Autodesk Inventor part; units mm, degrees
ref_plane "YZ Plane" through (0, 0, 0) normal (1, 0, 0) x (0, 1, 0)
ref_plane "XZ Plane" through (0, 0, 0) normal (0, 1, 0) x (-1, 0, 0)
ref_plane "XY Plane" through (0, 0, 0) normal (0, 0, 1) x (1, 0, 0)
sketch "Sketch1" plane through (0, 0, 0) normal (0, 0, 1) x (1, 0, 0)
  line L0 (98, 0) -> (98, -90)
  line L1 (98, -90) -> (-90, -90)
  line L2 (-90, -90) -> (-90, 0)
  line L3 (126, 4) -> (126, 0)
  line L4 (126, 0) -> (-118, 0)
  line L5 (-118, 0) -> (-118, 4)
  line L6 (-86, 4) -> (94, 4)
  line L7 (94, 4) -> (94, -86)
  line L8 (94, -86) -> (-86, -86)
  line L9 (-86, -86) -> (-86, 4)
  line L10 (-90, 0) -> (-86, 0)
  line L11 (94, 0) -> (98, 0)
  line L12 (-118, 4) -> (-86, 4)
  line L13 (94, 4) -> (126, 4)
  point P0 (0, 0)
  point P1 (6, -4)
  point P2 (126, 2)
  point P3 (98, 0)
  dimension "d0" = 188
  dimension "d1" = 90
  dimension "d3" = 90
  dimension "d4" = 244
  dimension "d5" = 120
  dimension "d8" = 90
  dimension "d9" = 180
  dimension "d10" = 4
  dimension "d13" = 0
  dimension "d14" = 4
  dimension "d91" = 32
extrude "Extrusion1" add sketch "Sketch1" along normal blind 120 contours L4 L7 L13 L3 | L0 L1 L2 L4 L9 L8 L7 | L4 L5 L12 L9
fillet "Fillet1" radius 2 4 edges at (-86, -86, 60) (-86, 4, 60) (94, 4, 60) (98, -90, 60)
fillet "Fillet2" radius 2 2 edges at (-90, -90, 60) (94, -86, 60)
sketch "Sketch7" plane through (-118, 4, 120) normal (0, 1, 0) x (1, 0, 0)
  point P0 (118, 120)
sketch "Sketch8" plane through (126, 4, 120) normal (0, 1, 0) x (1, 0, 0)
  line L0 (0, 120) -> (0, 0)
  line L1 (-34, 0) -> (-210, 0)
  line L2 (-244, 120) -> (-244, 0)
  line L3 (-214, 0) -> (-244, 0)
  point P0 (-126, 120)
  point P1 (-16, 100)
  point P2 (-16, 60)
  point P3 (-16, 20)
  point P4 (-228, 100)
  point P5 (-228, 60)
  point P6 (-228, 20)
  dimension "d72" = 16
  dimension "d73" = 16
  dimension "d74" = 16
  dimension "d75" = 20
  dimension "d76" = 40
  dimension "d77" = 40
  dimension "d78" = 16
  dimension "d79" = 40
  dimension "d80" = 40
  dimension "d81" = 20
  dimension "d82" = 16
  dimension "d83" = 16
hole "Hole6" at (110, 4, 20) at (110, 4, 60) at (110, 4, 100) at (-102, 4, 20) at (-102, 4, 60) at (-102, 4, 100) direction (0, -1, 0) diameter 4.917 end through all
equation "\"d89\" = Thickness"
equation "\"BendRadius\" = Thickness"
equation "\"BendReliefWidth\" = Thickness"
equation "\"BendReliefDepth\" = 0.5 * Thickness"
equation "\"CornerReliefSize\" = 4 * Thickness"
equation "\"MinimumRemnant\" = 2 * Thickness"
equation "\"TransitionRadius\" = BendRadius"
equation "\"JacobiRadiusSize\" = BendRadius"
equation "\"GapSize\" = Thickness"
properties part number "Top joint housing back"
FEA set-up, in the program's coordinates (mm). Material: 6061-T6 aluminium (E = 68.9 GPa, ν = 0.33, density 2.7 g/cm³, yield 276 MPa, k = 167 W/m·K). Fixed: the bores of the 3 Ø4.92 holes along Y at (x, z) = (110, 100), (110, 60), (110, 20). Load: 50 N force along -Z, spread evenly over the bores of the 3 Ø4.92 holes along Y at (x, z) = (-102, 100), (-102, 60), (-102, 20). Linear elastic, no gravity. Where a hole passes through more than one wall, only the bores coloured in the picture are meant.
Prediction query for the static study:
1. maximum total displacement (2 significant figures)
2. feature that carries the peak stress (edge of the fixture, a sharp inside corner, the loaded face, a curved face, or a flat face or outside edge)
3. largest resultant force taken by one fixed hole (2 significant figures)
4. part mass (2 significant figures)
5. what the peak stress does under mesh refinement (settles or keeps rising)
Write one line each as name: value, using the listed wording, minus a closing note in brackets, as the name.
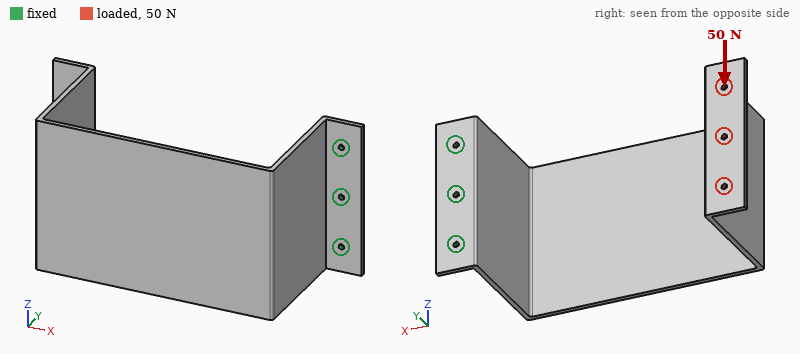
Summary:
maximum total displacement: 3.3 mm
feature that carries the peak stress: edge of the fixture
largest resultant force taken by one fixed hole: 130 N
part mass: 550 g
what the peak stress does under mesh refinement: keeps rising
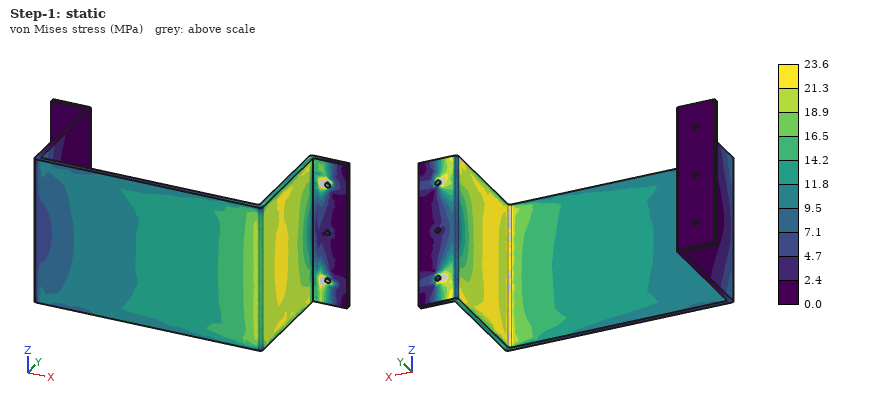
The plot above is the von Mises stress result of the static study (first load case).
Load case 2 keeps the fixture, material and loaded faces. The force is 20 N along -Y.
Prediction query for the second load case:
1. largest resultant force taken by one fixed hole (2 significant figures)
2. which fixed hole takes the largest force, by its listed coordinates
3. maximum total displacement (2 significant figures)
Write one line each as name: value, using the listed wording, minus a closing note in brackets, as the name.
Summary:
largest resultant force taken by one fixed hole: 21 N
which fixed hole takes the largest force, by its listed coordinates: (110, 60)
maximum total displacement: 3.3 mm
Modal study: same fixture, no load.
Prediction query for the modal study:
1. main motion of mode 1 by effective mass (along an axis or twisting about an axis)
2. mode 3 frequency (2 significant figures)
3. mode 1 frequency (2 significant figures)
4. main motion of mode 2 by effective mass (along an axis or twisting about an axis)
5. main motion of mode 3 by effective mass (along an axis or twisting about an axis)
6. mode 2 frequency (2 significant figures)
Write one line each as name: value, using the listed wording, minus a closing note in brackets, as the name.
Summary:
main motion of mode 1 by effective mass: along Y
mode 3 frequency: 95 Hz
mode 1 frequency: 29 Hz
main motion of mode 2 by effective mass: along Z
main motion of mode 3 by effective mass: along X
mode 2 frequency: 53 Hz
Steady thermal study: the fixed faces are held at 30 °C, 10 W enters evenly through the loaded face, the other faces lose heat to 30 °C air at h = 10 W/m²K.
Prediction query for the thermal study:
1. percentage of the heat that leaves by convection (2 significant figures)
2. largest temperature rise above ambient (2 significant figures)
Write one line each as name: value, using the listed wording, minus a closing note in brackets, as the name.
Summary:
percentage of the heat that leaves by convection: 80 %
largest temperature rise above ambient: 21 K
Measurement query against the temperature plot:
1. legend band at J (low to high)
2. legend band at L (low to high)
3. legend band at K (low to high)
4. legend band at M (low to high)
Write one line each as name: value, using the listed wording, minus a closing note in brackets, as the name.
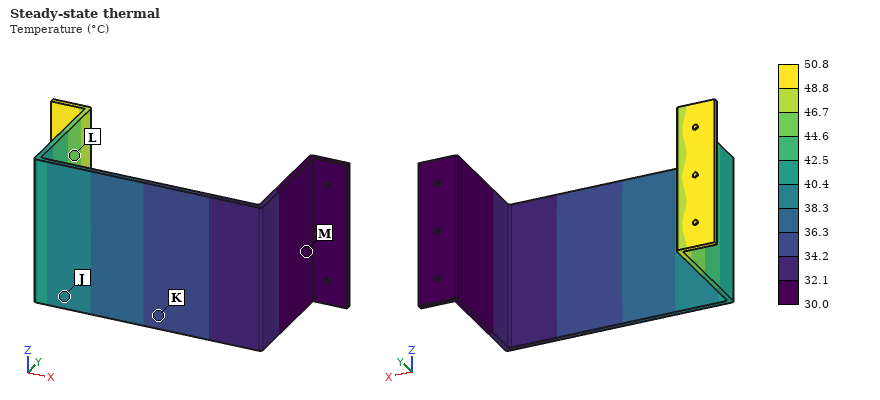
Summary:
legend band at J: 38.3 to 40.4 °C
legend band at L: 44.6 to 46.7 °C
legend band at K: 34.2 to 36.3 °C
legend band at M: 30.0 to 32.1 °C
